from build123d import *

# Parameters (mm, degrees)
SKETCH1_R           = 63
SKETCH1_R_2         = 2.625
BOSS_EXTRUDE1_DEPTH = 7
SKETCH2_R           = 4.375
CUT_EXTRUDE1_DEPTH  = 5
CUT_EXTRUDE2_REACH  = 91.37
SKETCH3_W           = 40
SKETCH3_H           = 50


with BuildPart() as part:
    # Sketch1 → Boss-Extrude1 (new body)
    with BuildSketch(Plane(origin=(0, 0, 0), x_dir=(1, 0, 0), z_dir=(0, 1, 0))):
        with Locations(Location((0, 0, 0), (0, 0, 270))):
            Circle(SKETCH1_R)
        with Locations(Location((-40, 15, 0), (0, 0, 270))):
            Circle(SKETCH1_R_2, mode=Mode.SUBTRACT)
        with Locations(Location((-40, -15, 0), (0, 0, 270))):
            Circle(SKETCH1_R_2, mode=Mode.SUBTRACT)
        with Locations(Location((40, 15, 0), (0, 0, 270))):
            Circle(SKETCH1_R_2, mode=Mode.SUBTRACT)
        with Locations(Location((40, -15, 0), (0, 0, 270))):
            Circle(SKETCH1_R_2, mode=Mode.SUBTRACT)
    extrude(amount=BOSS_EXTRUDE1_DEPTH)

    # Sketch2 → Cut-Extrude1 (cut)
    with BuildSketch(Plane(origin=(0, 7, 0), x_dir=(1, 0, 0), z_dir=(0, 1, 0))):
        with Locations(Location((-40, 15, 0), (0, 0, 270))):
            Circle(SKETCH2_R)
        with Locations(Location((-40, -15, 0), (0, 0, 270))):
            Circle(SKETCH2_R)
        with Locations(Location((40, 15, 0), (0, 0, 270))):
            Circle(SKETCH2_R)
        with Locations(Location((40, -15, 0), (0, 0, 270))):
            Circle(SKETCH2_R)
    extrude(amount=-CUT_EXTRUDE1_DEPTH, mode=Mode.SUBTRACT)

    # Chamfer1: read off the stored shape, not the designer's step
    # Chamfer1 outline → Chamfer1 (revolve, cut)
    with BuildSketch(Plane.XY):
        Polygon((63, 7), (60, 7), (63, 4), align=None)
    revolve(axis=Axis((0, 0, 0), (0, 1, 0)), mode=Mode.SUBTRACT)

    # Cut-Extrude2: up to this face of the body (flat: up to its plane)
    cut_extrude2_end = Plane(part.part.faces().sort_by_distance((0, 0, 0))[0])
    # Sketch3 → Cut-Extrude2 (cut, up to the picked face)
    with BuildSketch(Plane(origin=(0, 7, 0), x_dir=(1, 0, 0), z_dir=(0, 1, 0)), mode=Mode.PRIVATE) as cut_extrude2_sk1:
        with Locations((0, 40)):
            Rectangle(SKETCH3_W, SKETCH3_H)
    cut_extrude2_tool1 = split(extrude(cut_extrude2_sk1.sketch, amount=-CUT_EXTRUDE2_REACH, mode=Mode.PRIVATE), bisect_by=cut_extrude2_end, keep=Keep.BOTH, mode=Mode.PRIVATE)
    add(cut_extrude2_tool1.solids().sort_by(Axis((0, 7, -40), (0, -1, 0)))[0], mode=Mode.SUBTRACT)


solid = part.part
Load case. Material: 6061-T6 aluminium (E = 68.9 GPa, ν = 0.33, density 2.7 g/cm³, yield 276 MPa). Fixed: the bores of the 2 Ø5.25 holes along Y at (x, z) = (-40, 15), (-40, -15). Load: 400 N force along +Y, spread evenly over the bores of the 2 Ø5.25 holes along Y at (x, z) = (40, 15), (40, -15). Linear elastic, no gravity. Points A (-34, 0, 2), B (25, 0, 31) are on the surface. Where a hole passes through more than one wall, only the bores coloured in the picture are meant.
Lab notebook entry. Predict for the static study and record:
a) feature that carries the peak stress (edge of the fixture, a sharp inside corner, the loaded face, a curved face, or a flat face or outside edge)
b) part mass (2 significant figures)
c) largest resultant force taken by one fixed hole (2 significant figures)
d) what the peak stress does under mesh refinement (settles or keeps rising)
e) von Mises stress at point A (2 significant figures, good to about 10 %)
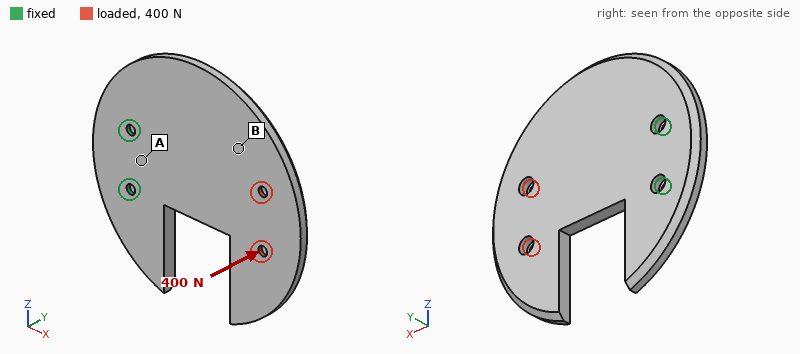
edge of the fixture
190 g
400 N
keeps rising
55 MPa
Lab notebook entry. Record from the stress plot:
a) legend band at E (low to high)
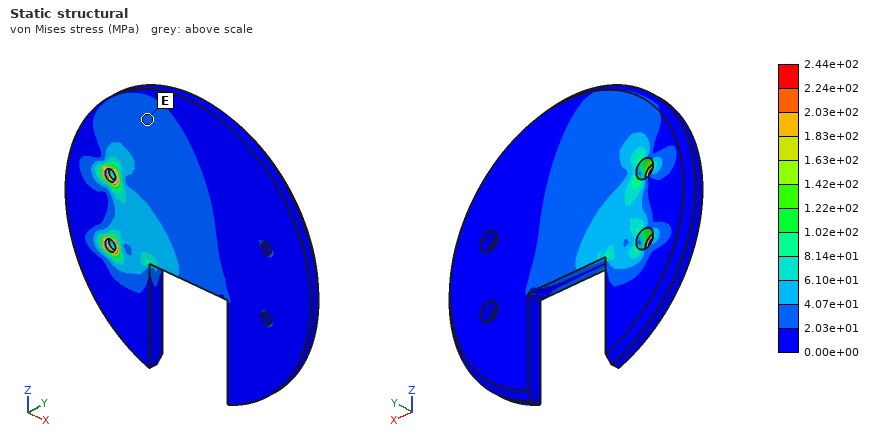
2.03e+01 to 4.07e+01 MPa
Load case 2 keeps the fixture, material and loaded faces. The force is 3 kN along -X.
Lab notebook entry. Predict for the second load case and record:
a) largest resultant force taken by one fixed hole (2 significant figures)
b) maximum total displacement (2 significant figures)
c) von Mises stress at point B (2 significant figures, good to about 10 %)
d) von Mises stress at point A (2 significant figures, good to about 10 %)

1.5 kN
0.26 mm
13 MPa
16 MPa
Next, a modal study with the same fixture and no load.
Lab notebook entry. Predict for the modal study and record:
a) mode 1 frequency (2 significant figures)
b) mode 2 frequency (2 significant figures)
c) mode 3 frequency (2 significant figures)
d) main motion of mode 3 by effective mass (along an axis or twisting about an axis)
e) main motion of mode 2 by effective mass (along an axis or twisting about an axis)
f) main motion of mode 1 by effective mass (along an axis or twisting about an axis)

330 Hz
920 Hz
2000 Hz
along Z
twisting about X
along Y
